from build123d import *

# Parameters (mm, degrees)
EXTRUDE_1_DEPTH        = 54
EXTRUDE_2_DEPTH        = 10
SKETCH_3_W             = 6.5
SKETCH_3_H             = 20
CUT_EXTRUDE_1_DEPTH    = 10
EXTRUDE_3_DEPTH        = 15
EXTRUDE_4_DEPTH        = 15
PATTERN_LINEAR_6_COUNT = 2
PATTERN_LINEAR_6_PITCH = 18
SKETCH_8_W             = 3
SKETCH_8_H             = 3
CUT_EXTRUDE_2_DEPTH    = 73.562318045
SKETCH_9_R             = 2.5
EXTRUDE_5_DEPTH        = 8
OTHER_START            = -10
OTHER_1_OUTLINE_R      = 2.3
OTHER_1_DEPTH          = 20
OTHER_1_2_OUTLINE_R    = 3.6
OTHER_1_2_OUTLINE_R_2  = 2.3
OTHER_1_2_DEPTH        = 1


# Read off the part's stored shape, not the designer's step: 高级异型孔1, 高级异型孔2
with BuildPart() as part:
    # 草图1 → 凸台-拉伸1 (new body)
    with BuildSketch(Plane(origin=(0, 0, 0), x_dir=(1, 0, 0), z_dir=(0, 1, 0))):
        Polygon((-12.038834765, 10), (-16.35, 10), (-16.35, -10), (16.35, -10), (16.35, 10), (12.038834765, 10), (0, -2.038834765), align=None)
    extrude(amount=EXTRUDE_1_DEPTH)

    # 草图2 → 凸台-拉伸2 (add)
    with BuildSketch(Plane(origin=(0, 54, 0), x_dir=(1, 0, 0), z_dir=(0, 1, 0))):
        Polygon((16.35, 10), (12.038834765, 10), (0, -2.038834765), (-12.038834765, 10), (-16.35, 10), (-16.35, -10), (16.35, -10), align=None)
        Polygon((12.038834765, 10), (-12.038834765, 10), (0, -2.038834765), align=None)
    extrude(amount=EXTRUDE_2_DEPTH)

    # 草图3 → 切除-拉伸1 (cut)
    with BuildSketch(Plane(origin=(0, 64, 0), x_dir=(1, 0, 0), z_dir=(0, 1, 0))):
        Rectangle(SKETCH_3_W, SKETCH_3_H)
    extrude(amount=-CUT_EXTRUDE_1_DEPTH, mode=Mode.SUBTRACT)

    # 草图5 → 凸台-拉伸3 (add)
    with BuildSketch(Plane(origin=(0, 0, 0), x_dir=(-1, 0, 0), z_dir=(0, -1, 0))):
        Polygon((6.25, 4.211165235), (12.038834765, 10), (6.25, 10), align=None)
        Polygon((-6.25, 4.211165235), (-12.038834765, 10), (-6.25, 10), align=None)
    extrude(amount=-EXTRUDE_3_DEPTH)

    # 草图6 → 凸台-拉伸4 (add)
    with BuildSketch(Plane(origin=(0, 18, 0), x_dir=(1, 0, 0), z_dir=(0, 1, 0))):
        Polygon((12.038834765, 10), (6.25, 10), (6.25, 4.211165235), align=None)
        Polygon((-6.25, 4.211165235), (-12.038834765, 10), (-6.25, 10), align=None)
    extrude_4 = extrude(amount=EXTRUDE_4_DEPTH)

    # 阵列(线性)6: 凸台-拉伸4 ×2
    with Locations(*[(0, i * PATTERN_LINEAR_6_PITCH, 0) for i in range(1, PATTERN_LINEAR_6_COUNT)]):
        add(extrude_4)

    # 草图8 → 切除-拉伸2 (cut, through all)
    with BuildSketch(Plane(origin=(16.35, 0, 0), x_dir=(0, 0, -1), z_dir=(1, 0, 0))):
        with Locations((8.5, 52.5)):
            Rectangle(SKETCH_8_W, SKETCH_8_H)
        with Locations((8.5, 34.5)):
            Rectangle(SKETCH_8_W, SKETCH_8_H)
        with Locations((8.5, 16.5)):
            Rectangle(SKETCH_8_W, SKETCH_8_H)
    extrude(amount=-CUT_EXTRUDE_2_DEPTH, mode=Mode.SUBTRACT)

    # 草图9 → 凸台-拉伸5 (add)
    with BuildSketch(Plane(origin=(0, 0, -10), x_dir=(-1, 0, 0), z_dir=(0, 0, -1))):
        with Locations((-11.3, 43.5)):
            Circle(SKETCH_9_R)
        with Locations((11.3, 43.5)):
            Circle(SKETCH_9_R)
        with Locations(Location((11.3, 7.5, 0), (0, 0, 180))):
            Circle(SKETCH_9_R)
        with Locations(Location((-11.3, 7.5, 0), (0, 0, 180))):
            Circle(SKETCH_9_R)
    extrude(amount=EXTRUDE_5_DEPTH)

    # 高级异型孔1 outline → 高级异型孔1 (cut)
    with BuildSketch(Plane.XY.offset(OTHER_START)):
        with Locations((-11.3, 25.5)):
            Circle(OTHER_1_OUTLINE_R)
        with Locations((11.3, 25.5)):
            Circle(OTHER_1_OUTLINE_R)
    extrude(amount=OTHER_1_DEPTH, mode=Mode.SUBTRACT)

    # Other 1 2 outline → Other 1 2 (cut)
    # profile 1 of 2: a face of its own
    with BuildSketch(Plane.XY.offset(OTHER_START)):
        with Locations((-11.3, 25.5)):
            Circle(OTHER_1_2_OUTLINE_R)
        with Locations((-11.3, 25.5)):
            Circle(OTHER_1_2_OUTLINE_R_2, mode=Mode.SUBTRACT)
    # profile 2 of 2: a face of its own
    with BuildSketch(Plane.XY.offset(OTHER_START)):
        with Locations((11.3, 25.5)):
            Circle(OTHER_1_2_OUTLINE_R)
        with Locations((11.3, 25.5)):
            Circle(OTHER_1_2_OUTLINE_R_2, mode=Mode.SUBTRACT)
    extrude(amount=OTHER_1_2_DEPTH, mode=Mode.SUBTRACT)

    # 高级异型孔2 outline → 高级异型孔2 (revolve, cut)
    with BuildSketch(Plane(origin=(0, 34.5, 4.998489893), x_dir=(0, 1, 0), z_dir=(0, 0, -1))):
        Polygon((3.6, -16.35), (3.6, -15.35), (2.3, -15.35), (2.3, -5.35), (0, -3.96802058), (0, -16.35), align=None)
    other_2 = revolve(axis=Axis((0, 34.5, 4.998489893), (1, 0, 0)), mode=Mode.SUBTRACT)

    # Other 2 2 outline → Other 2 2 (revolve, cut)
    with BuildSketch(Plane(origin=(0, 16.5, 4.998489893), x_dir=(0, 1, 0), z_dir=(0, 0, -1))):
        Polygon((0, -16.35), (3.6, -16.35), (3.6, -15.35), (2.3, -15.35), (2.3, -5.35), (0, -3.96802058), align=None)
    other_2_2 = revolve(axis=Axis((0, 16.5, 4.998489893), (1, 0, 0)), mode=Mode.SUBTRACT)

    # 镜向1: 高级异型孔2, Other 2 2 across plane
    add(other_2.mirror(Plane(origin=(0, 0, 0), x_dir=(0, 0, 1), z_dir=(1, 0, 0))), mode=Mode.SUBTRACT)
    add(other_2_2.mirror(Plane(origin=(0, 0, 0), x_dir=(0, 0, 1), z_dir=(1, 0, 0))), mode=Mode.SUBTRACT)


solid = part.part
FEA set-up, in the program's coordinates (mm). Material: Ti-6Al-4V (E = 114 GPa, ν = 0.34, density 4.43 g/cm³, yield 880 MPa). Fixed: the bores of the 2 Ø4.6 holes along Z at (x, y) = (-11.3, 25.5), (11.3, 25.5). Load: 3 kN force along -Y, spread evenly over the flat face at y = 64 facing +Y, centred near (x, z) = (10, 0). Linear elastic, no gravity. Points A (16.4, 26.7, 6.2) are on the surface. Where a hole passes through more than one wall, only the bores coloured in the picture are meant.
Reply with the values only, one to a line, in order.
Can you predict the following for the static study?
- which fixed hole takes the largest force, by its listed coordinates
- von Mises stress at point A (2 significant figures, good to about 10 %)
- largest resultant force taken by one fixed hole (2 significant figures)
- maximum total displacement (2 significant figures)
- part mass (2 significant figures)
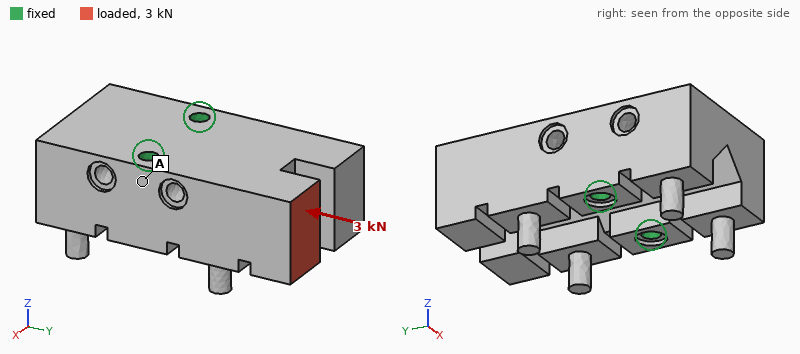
(11.3, 25.5)
4.6 MPa
2.7 kN
8.8 µm
150 g
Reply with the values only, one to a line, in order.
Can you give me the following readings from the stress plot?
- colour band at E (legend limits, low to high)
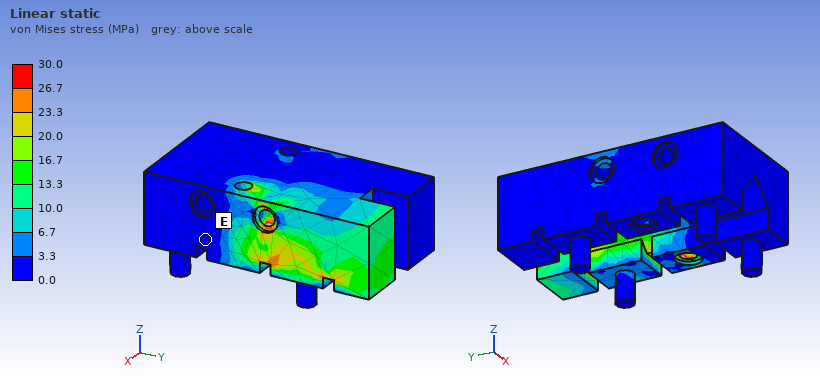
0.0 to 3.3 MPa
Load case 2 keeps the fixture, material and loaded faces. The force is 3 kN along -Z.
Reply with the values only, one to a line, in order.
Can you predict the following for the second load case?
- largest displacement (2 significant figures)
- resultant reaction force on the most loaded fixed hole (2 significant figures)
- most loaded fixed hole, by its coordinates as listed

87 µm
2.4 kN
(11.3, 25.5)
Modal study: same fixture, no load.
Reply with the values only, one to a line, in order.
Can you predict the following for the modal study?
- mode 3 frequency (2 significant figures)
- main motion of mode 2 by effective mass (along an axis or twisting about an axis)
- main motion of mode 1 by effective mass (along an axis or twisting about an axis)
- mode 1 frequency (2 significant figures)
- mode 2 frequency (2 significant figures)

13 kHz
along X
along Z
7800 Hz
8900 Hz
